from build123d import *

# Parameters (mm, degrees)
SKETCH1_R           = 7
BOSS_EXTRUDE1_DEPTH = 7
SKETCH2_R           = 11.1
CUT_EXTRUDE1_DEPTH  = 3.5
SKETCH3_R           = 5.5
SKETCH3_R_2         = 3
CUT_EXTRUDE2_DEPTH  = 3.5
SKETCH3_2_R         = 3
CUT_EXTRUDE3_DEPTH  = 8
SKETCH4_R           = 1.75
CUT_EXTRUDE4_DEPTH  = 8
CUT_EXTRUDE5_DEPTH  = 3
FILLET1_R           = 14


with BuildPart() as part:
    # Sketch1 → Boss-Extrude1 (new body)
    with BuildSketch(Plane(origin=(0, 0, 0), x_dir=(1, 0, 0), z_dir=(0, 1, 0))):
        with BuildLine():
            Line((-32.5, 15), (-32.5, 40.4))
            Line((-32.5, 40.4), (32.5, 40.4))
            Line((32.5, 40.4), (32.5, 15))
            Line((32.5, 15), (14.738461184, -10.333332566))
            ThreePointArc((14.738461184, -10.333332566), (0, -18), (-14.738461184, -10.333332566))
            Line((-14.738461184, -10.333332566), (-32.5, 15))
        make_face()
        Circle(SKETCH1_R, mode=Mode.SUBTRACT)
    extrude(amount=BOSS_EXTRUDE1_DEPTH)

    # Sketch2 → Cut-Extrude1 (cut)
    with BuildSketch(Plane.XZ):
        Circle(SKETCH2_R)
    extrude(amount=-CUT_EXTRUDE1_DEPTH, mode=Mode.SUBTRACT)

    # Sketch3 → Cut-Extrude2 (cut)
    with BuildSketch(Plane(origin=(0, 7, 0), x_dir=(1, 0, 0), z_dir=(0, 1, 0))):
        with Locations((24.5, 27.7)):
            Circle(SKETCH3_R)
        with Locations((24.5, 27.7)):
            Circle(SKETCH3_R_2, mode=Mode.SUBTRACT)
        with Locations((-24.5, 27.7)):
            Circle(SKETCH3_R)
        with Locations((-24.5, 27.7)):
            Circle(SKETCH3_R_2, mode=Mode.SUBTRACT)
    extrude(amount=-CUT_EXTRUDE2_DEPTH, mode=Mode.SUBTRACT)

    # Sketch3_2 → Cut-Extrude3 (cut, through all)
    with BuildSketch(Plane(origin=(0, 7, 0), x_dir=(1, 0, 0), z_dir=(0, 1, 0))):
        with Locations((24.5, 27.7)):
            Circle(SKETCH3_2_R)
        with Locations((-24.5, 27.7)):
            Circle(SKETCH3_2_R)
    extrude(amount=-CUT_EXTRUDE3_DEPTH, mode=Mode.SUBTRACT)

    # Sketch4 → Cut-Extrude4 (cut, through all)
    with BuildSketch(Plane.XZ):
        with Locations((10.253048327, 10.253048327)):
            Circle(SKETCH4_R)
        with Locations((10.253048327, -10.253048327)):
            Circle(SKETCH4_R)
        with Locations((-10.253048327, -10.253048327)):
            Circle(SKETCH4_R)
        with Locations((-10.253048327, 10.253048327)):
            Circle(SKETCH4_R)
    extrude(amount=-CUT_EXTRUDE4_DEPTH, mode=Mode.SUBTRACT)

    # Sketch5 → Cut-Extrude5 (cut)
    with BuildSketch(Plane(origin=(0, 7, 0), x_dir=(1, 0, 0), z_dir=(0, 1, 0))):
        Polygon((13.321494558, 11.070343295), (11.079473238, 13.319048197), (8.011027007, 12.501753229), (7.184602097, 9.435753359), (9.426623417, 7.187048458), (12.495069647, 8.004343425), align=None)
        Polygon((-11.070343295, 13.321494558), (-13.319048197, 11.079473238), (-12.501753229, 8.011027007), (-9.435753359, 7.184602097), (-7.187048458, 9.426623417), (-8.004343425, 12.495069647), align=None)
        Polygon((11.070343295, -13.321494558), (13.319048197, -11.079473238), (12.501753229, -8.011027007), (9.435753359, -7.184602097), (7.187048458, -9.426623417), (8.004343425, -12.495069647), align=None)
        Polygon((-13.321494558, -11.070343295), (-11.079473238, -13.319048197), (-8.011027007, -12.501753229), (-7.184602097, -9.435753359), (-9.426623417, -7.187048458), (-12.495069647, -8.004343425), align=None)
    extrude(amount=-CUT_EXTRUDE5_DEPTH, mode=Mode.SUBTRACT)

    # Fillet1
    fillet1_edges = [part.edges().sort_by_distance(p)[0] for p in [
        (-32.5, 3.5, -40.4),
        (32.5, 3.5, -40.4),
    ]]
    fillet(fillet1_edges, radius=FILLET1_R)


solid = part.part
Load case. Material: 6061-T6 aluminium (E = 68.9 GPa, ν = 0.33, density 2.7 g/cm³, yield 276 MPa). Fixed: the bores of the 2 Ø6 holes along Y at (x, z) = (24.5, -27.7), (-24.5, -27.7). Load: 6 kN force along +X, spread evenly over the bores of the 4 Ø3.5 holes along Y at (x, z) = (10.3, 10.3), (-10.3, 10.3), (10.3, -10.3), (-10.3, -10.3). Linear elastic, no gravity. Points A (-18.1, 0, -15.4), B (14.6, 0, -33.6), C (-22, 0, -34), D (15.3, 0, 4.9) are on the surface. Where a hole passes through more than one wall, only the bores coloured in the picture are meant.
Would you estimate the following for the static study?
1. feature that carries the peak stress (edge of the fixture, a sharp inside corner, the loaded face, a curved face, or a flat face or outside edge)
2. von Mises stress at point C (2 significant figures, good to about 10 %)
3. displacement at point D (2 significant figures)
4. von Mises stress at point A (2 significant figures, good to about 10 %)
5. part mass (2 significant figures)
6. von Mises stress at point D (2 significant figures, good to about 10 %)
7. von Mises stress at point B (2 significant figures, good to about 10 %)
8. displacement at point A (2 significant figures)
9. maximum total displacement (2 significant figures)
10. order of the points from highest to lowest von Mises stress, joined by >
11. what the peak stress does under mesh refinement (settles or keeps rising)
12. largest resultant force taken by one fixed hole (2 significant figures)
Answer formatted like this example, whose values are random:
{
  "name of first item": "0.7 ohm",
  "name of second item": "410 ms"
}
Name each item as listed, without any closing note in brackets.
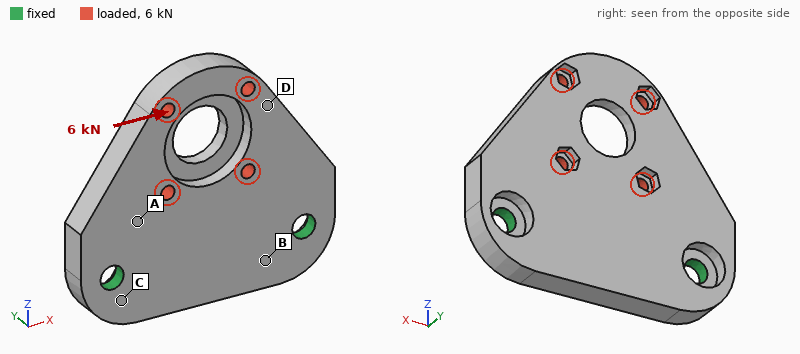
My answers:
{
  "feature that carries the peak stress": "edge of the fixture",
  "von Mises stress at point C": "27 MPa",
  "displacement at point D": "69 µm",
  "von Mises stress at point A": "48 MPa",
  "part mass": "47 g",
  "von Mises stress at point D": "68 MPa",
  "von Mises stress at point B": "13 MPa",
  "displacement at point A": "21 µm",
  "maximum total displacement": "92 µm",
  "order of the points from highest to lowest von Mises stress, joined by >": "D > A > C > B",
  "what the peak stress does under mesh refinement": "keeps rising",
  "largest resultant force taken by one fixed hole": "4.4 kN"
}
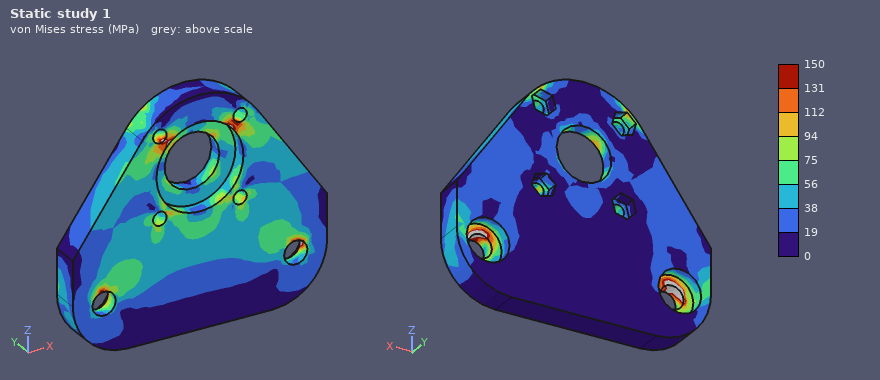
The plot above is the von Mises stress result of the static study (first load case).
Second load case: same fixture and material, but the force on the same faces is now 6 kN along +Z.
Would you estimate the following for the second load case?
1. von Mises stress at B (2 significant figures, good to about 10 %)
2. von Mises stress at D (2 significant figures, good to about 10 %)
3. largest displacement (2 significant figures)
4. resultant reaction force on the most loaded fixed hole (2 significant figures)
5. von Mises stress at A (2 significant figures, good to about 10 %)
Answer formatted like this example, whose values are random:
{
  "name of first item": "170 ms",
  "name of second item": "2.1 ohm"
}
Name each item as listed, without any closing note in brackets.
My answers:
{
  "von Mises stress at B": "17 MPa",
  "von Mises stress at D": "58 MPa",
  "largest displacement": "81 µm",
  "resultant reaction force on the most loaded fixed hole": "3.1 kN",
  "von Mises stress at A": "43 MPa"
}
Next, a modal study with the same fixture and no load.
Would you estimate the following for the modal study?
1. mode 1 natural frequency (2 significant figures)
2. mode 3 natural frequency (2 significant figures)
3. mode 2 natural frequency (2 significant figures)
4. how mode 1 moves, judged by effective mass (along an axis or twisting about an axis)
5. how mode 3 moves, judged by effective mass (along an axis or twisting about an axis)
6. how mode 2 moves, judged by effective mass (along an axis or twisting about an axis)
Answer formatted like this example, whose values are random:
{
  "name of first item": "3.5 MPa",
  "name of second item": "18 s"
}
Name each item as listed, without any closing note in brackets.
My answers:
{
  "mode 1 natural frequency": "2700 Hz",
  "mode 3 natural frequency": "10 kHz",
  "mode 2 natural frequency": "7700 Hz",
  "how mode 1 moves, judged by effective mass": "along Y",
  "how mode 3 moves, judged by effective mass": "along Y",
  "how mode 2 moves, judged by effective mass": "twisting about Z"
}
